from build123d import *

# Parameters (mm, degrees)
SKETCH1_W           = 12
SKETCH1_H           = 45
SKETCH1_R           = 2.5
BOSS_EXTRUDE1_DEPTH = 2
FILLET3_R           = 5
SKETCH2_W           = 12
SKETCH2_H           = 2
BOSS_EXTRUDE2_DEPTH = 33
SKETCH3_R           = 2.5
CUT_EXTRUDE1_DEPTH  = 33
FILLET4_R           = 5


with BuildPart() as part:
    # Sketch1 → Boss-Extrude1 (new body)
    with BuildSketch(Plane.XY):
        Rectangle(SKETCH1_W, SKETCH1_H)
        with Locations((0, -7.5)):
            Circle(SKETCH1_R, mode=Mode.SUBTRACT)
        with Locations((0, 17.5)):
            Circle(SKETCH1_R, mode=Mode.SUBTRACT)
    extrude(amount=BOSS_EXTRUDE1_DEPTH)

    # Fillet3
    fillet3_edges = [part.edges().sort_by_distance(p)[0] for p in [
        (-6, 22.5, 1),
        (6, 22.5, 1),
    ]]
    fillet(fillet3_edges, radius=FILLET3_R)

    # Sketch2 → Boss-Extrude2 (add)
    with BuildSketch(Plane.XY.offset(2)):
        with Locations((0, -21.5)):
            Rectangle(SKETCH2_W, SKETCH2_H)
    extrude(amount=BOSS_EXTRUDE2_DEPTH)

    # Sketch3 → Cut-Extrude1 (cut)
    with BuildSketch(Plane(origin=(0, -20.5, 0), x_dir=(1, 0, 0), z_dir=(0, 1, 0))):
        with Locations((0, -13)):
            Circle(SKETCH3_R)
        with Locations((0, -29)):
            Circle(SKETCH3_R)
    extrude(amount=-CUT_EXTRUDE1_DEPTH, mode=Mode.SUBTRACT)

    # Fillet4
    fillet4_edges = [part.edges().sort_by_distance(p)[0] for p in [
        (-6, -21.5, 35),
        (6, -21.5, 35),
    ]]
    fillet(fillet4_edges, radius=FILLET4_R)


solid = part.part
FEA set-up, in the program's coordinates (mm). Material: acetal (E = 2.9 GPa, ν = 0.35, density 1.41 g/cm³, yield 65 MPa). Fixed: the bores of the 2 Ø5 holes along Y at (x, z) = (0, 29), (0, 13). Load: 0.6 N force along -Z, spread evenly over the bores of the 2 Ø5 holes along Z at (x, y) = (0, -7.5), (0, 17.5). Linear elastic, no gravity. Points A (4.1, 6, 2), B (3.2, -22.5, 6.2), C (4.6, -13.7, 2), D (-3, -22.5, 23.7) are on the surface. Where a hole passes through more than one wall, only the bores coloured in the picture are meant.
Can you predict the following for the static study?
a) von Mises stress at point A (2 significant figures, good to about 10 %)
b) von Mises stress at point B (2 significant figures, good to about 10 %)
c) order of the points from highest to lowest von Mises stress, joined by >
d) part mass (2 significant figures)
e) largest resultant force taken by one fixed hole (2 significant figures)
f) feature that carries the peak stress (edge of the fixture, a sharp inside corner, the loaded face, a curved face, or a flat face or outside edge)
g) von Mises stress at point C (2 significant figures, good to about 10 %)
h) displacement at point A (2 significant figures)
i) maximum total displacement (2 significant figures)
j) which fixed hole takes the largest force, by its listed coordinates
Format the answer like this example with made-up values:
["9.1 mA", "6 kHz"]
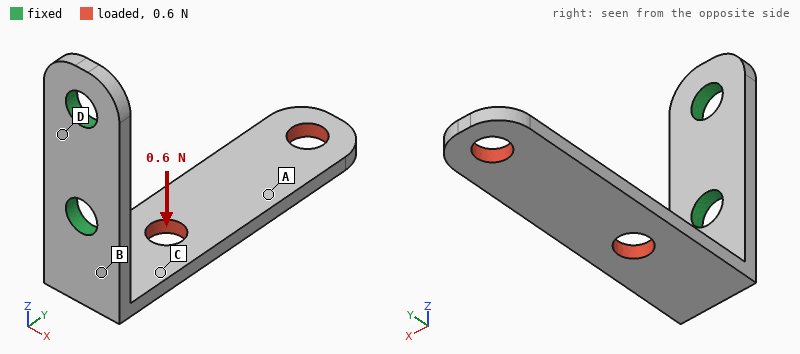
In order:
["0.44 MPa", "1.8 MPa", "B > C > A > D", "2.4 g", "0.57 N", "a flat face or outside edge", "1.4 MPa", "0.36 mm", "0.66 mm", "(0, 13)"]
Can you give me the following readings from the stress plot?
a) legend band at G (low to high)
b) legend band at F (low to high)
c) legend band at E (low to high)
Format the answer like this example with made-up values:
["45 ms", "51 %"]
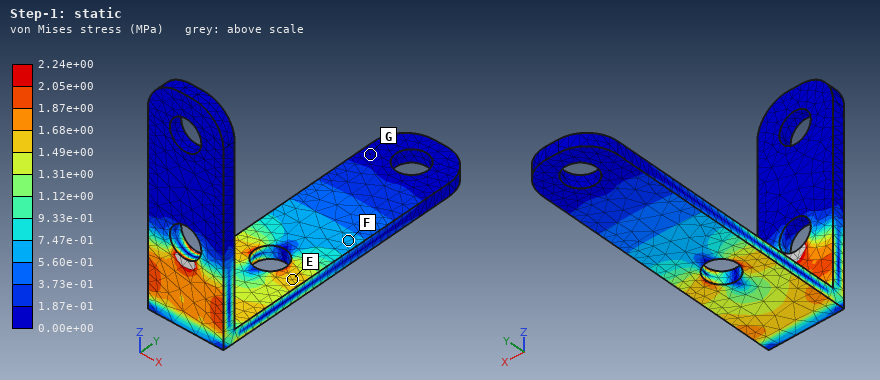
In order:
["0.00e+00 to 1.87e-01 MPa", "5.60e-01 to 7.47e-01 MPa", "1.49e+00 to 1.68e+00 MPa"]
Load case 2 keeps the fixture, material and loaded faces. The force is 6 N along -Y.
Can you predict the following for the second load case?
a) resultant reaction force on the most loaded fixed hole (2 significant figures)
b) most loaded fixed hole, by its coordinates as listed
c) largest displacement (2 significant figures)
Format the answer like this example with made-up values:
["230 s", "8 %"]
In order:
["6.0 N", "(0, 13)", "0.58 mm"]
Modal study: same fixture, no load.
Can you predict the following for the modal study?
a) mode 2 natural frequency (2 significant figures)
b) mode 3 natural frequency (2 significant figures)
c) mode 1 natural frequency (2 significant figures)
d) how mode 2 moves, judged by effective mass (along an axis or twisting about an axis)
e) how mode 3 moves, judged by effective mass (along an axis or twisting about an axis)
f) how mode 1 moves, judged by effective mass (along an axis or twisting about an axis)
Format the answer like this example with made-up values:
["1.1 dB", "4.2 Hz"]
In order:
["350 Hz", "1100 Hz", "190 Hz", "along X", "along Y", "along Z"]
